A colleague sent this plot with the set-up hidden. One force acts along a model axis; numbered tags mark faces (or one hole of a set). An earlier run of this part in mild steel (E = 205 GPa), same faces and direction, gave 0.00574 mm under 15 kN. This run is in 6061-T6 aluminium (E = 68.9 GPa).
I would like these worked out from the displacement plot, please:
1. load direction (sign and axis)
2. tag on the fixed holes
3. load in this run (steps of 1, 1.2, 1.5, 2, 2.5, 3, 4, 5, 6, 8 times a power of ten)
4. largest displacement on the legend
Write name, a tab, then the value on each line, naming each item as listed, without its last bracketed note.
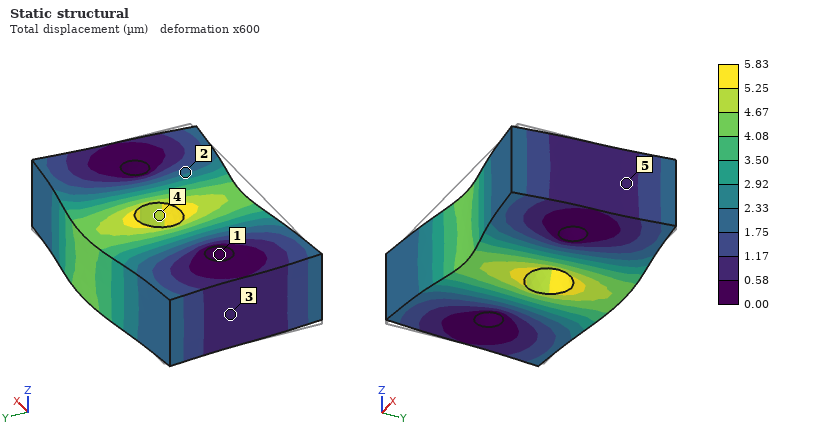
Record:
load direction	+Y
tag on the fixed holes	1
load in this run	5 kN
largest displacement on the legend	5.83 µm
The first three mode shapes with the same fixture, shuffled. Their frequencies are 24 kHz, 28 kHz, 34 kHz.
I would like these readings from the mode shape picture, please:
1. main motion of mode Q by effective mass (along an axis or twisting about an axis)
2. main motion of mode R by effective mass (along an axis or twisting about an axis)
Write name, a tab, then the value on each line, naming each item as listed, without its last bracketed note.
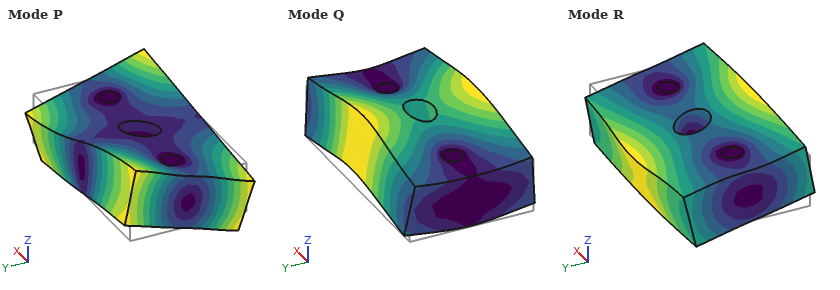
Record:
main motion of mode Q by effective mass	along Z
main motion of mode R by effective mass	twisting about X
